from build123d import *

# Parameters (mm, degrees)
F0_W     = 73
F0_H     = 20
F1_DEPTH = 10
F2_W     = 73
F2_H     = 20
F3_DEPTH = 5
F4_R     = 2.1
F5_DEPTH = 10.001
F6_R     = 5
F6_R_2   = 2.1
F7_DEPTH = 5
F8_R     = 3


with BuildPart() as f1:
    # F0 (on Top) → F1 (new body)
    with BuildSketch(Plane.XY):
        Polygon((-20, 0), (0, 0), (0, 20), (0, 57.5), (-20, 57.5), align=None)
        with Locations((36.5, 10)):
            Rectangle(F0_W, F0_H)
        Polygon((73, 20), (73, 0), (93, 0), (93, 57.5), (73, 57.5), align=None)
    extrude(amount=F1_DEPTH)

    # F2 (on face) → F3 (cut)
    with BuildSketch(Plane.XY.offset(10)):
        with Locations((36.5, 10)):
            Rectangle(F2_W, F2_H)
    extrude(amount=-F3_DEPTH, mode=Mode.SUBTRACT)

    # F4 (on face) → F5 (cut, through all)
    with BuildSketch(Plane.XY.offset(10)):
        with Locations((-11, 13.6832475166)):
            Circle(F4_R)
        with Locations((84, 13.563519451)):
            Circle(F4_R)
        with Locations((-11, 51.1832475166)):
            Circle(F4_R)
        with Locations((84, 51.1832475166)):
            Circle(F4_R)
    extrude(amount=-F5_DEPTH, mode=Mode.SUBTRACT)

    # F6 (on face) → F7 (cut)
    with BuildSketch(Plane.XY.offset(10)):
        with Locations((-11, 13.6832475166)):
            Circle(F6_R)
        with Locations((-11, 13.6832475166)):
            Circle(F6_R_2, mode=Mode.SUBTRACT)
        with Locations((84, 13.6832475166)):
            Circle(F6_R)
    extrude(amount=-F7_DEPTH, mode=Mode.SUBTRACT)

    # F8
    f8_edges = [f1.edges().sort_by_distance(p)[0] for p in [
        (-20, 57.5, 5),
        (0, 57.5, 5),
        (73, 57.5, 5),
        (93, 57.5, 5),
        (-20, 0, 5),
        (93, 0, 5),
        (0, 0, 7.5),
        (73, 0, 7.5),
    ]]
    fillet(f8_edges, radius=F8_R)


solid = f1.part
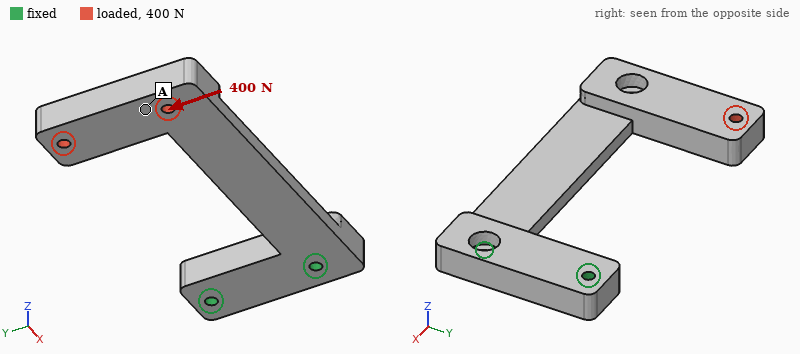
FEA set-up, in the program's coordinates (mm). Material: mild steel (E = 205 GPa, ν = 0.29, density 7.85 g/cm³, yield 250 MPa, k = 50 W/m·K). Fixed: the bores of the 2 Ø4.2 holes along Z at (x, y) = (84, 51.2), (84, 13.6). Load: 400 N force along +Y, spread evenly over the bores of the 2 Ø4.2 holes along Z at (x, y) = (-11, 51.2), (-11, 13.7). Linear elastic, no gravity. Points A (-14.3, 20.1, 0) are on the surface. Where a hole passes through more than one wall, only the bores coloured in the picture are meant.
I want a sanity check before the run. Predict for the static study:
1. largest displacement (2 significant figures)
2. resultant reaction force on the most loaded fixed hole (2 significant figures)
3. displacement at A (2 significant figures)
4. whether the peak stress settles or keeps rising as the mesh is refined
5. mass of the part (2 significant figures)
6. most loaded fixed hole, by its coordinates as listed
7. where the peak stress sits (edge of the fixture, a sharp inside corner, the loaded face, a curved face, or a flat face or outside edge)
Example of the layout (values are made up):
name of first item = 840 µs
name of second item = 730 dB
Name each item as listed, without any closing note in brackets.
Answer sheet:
largest displacement = 0.25 mm
resultant reaction force on the most loaded fixed hole = 1.1 kN
displacement at A = 0.19 mm
whether the peak stress settles or keeps rising as the mesh is refined = keeps rising
mass of the part = 230 g
most loaded fixed hole, by its coordinates as listed = (84, 51.2)
where the peak stress sits = edge of the fixture
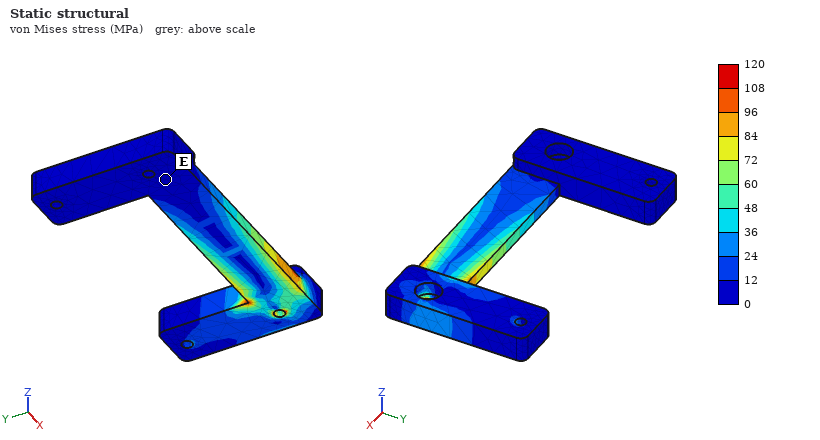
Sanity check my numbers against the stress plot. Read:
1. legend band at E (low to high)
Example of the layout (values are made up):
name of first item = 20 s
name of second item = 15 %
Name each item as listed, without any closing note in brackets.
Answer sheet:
legend band at E = 0 to 12 MPa
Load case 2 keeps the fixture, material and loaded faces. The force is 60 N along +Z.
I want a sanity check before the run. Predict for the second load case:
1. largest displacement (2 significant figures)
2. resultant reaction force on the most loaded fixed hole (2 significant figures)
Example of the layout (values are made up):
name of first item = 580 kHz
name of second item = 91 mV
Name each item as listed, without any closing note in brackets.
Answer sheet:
largest displacement = 0.48 mm
resultant reaction force on the most loaded fixed hole = 59 N
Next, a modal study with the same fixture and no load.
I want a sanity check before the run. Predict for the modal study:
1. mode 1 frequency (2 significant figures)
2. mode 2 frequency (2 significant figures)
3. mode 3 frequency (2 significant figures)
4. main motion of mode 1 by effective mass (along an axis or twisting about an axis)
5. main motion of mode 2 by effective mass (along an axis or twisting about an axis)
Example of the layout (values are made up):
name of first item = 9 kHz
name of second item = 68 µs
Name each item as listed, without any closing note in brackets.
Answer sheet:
mode 1 frequency = 220 Hz
mode 2 frequency = 720 Hz
mode 3 frequency = 870 Hz
main motion of mode 1 by effective mass = along Z
main motion of mode 2 by effective mass = along Y
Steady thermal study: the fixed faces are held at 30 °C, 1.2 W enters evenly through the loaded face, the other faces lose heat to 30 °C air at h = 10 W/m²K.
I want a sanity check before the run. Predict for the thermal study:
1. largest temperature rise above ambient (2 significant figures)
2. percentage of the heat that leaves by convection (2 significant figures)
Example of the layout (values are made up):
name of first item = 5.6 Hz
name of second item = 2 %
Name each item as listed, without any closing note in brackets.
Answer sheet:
largest temperature rise above ambient = 13 K
percentage of the heat that leaves by convection = 54 %
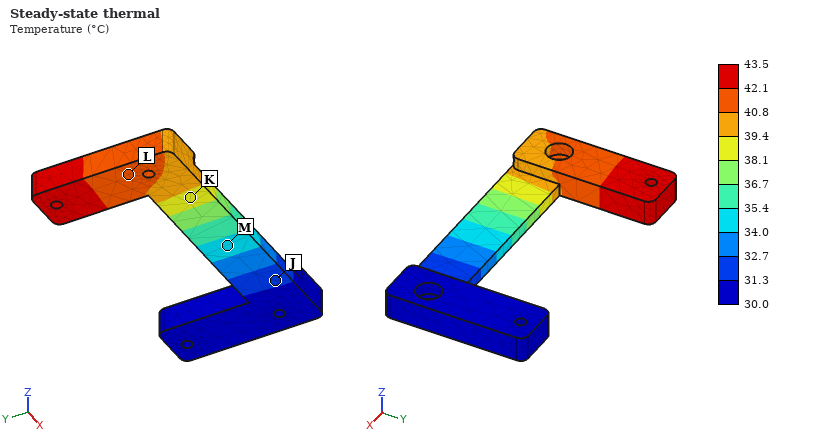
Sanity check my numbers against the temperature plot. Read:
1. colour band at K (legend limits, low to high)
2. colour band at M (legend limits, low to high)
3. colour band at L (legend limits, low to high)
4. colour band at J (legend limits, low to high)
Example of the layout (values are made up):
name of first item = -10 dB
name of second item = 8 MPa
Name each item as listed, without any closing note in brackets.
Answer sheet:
colour band at K = 38.1 to 39.4 °C
colour band at M = 34.0 to 35.4 °C
colour band at L = 40.8 to 42.1 °C
colour band at J = 31.3 to 32.7 °C
